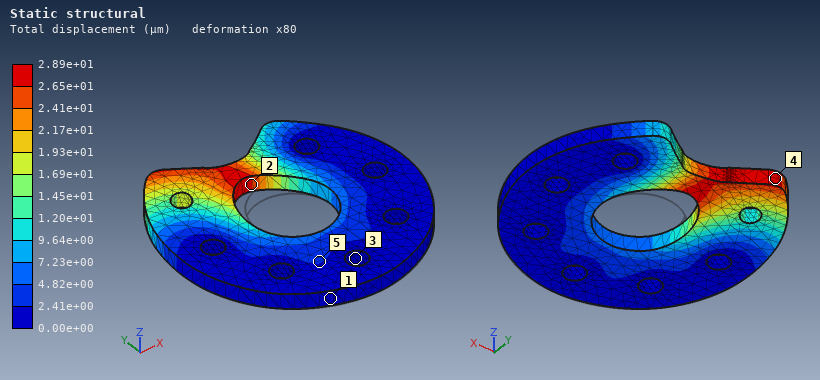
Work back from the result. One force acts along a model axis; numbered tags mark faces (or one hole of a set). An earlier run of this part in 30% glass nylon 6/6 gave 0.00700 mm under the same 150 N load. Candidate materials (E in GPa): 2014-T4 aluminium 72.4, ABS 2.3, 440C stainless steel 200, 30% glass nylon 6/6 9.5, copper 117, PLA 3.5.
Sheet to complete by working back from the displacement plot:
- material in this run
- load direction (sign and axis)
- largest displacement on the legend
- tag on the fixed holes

ABS
+Y
2.89e+01 µm
3
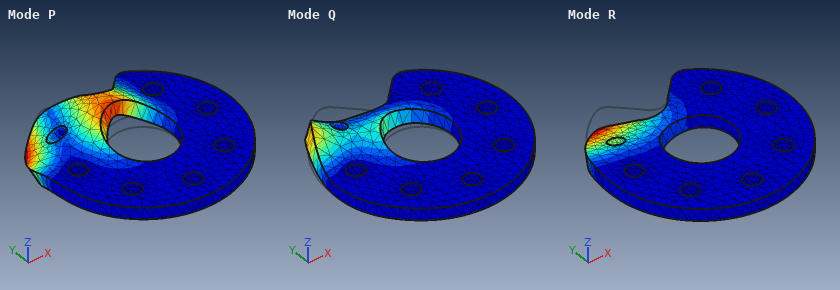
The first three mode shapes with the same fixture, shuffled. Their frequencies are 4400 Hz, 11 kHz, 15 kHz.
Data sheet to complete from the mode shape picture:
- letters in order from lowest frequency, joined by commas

R, P, Q
